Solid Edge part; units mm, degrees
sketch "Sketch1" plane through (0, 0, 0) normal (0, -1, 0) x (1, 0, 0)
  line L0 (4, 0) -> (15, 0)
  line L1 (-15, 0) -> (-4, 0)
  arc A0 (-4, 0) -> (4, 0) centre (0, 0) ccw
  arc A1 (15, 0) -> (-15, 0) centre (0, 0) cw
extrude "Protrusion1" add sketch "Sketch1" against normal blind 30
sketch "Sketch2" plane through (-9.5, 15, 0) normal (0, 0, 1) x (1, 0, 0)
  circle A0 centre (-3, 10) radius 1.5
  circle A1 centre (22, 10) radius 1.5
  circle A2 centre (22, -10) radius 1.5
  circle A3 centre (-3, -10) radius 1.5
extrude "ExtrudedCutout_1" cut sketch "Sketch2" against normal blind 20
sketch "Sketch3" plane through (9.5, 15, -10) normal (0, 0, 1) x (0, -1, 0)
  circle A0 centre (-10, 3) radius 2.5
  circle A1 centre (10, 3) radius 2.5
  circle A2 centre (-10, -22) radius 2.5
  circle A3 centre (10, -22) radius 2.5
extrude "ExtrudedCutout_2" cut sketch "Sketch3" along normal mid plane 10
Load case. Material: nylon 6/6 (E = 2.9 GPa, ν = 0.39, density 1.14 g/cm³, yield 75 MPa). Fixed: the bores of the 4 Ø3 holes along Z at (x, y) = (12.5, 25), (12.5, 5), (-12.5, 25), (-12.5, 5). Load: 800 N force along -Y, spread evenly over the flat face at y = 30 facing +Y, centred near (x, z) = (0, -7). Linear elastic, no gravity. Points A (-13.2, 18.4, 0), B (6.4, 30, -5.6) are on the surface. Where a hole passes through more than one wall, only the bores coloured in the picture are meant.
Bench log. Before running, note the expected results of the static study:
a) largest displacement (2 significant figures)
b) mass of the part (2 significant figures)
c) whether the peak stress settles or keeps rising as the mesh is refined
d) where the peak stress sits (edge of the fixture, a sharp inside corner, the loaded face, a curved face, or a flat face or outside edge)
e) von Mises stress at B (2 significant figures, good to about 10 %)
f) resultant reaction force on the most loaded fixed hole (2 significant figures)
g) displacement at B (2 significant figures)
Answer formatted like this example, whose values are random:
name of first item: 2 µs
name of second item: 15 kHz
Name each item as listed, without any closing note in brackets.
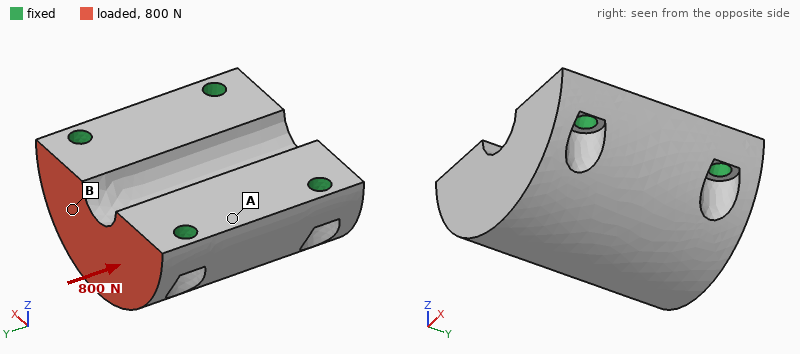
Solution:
largest displacement: 41 µm
mass of the part: 11 g
whether the peak stress settles or keeps rising as the mesh is refined: keeps rising
where the peak stress sits: edge of the fixture
von Mises stress at B: 3.0 MPa
resultant reaction force on the most loaded fixed hole: 270 N
displacement at B: 26 µm
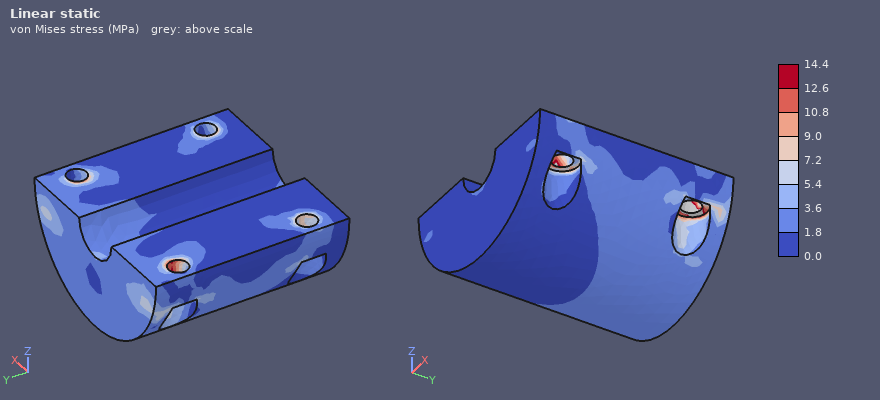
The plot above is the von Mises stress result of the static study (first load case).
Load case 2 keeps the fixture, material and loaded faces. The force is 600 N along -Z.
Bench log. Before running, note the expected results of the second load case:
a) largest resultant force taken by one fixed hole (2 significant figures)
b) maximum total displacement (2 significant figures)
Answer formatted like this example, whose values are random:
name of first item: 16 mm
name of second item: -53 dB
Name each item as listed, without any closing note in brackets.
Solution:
largest resultant force taken by one fixed hole: 380 N
maximum total displacement: 71 µm
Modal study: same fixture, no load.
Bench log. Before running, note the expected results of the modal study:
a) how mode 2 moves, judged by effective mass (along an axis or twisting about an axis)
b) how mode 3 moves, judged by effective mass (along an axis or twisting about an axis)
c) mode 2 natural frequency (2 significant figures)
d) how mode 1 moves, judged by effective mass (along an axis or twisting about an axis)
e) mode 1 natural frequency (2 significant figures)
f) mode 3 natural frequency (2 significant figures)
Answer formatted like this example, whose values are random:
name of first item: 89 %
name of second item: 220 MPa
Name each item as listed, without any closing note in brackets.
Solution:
how mode 2 moves, judged by effective mass: along Z
how mode 3 moves, judged by effective mass: along X
mode 2 natural frequency: 10 kHz
how mode 1 moves, judged by effective mass: along Y
mode 1 natural frequency: 9300 Hz
mode 3 natural frequency: 12 kHz
